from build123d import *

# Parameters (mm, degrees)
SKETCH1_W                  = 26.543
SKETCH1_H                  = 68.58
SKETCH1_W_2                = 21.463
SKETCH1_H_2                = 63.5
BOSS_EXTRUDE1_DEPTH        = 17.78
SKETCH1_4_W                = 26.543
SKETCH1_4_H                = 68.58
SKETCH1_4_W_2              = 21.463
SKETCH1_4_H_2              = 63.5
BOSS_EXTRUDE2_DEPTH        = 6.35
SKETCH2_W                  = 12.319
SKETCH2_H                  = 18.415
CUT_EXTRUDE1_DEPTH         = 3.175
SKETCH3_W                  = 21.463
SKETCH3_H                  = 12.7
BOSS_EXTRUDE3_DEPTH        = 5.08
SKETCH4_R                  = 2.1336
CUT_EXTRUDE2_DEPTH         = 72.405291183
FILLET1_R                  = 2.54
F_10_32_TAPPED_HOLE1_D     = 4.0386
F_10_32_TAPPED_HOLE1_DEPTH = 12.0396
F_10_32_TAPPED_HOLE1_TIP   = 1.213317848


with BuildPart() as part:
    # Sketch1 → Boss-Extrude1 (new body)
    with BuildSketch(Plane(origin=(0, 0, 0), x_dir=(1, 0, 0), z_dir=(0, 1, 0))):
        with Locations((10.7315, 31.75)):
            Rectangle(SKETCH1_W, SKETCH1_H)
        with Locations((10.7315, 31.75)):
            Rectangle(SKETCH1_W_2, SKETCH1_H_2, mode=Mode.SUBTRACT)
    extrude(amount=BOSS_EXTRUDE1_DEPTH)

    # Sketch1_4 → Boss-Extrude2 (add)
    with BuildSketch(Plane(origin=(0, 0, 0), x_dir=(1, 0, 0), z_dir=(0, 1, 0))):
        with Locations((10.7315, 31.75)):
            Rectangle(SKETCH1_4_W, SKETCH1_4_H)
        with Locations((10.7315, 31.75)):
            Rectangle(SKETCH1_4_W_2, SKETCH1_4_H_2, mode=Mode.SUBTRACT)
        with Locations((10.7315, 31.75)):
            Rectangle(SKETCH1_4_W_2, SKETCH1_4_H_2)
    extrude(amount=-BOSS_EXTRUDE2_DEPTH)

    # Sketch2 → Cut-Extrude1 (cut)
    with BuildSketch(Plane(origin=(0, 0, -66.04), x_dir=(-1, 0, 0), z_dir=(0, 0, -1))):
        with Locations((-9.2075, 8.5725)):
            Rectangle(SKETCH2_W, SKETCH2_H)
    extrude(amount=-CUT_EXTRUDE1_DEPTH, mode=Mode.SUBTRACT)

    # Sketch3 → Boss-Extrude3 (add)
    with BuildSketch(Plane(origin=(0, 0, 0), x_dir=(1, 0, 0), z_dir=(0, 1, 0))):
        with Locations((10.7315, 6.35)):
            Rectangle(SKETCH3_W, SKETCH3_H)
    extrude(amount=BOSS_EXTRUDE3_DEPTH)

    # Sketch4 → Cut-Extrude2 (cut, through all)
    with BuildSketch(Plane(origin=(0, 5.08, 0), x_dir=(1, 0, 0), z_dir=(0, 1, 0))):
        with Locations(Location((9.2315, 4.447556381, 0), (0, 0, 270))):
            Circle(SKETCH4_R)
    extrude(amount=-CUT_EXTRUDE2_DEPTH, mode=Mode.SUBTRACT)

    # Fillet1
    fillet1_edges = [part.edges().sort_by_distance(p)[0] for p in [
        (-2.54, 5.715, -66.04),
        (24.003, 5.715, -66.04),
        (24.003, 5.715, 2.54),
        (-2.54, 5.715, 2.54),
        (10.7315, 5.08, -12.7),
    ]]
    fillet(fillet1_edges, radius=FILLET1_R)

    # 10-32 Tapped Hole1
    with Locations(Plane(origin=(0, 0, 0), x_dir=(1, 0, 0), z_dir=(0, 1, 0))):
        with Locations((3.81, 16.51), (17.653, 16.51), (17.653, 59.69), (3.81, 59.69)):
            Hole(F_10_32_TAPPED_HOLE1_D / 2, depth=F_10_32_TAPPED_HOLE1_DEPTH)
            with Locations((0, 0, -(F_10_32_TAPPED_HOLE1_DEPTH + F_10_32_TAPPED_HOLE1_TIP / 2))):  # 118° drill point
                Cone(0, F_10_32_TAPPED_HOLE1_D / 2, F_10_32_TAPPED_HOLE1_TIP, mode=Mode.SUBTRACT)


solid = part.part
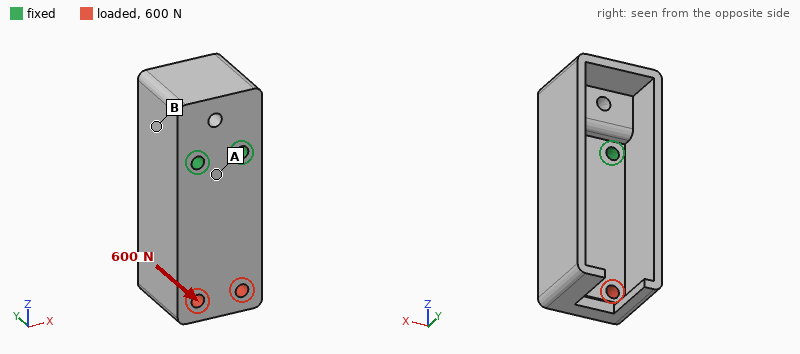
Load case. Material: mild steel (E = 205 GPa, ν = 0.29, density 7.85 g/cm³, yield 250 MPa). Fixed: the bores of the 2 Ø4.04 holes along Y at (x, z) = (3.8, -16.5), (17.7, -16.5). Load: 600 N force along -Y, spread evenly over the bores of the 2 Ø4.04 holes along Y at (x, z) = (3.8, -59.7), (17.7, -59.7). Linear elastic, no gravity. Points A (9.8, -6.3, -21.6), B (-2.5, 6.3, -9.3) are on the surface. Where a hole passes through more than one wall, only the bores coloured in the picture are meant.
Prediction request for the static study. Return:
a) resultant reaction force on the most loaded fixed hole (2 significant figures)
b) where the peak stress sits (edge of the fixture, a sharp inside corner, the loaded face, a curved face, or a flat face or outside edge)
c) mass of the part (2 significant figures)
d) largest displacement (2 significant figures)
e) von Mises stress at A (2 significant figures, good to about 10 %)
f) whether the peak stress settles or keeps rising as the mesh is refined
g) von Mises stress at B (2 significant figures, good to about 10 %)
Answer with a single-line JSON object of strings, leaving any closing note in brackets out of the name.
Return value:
{"resultant reaction force on the most loaded fixed hole": "300 N", "where the peak stress sits": "edge of the fixture", "mass of the part": "160 g", "largest displacement": "43 µm", "von Mises stress at A": "33 MPa", "whether the peak stress settles or keeps rising as the mesh is refined": "keeps rising", "von Mises stress at B": "12 MPa"}
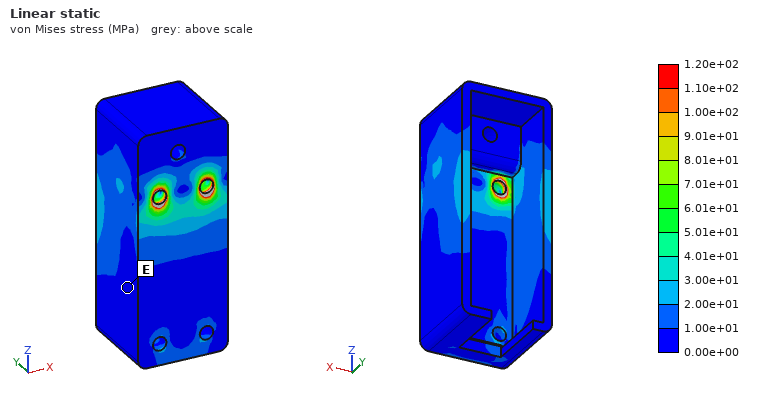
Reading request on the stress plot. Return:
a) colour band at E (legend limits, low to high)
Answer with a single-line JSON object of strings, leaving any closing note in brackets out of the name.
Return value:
{"colour band at E": "0.00e+00 to 1.00e+01 MPa"}
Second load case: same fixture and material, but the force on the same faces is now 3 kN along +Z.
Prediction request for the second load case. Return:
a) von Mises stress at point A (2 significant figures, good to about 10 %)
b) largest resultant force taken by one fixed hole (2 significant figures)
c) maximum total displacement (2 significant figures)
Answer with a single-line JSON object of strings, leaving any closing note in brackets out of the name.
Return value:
{"von Mises stress at point A": "14 MPa", "largest resultant force taken by one fixed hole": "1.5 kN", "maximum total displacement": "7.0 µm"}
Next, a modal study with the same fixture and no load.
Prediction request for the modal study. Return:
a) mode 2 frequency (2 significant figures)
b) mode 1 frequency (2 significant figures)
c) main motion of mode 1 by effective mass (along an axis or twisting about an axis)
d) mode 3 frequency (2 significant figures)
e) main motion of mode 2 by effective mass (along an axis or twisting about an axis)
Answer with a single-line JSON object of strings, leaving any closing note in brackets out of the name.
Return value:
{"mode 2 frequency": "4000 Hz", "mode 1 frequency": "3000 Hz", "main motion of mode 1 by effective mass": "along Y", "mode 3 frequency": "6500 Hz", "main motion of mode 2 by effective mass": "along X"}
